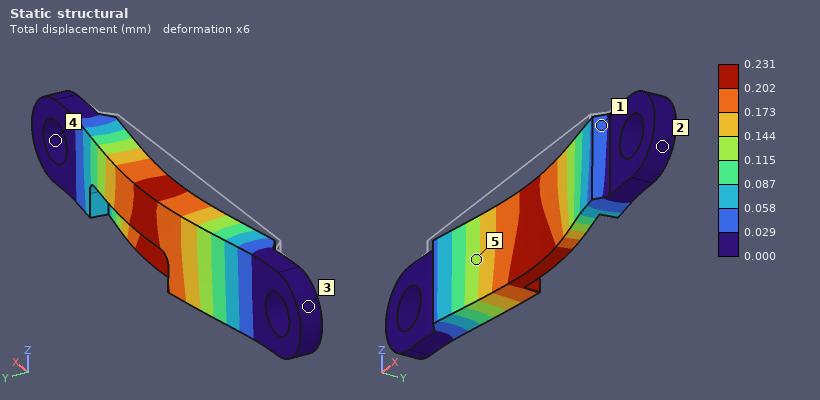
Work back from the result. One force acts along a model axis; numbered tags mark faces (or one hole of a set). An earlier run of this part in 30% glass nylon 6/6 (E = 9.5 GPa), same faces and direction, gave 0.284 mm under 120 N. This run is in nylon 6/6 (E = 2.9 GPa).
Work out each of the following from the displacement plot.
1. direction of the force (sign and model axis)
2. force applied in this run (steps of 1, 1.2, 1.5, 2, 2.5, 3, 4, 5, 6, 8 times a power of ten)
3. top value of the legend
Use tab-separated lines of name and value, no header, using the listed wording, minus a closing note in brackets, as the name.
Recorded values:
direction of the force	+Y
force applied in this run	30 N
top value of the legend	0.231 mm
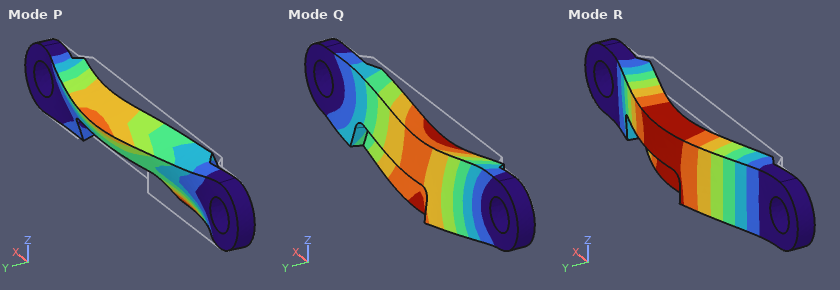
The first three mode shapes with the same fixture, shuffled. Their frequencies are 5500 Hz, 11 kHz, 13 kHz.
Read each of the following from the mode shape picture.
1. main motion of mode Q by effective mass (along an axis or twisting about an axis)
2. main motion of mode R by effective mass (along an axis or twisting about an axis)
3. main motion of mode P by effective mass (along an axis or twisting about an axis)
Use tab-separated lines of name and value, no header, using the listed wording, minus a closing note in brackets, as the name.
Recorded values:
main motion of mode Q by effective mass	along Z
main motion of mode R by effective mass	along Y
main motion of mode P by effective mass	twisting about X
